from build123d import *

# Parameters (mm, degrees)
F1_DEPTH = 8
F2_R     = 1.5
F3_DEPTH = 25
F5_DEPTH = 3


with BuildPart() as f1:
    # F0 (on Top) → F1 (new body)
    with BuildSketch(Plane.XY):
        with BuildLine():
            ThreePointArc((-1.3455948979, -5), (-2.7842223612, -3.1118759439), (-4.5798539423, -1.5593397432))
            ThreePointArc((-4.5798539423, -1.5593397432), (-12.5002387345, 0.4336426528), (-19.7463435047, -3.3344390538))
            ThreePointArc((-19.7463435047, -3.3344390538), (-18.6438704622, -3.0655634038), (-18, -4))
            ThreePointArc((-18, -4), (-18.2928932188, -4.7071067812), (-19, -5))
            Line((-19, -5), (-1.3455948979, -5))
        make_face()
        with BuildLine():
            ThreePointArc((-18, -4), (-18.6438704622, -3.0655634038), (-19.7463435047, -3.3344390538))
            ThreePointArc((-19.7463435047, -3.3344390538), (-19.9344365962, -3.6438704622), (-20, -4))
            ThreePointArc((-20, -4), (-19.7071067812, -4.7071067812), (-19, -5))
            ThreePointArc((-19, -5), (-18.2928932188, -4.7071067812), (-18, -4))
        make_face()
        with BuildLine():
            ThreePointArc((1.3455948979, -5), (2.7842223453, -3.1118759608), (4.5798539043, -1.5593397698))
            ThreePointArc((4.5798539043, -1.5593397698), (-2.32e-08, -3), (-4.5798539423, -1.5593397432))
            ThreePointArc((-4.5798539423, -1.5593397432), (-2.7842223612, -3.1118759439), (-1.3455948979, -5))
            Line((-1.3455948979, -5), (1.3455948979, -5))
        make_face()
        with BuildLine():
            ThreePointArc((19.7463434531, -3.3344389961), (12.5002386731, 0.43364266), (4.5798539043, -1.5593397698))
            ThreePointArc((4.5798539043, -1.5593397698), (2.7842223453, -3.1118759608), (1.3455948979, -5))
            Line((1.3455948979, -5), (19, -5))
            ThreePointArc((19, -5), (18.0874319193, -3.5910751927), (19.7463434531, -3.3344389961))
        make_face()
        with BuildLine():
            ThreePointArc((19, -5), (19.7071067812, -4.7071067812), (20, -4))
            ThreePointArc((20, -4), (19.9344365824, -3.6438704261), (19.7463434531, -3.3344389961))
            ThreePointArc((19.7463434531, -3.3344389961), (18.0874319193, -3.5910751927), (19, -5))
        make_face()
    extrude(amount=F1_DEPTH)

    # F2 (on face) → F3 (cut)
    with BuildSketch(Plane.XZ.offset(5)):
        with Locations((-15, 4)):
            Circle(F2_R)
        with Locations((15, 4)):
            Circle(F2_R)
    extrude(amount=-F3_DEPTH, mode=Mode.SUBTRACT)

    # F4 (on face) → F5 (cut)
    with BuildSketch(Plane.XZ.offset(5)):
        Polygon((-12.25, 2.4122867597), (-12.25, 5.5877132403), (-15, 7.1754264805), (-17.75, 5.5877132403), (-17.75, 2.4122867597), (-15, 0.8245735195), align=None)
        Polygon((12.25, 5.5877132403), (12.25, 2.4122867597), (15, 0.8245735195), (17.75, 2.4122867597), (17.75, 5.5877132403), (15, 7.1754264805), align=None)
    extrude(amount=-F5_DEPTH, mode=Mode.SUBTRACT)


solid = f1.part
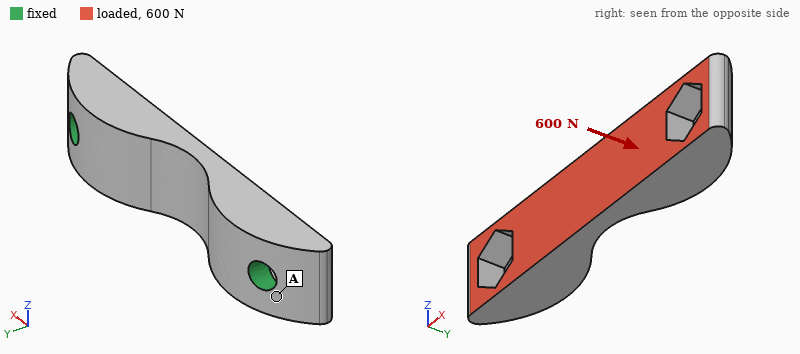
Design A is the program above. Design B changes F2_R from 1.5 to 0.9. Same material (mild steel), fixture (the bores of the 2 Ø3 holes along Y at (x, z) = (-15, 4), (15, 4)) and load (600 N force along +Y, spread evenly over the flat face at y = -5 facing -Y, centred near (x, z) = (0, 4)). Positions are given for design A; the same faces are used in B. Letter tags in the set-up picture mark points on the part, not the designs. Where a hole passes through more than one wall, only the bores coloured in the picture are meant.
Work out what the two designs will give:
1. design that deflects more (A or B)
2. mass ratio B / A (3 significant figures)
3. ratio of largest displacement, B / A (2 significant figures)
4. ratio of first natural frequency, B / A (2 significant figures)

B
1.01
1.4
0.76
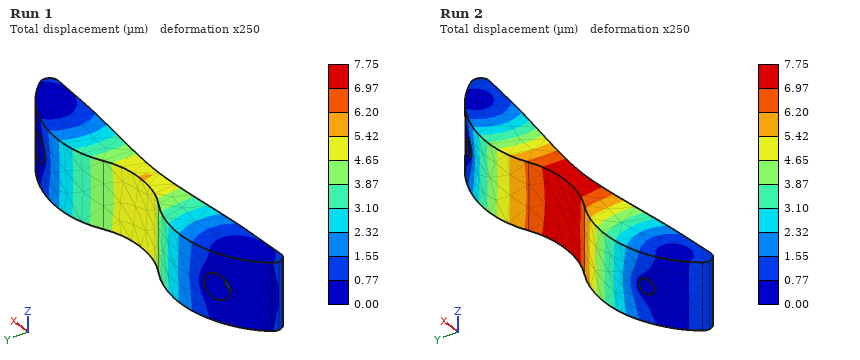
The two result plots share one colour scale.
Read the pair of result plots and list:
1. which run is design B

Run 2
